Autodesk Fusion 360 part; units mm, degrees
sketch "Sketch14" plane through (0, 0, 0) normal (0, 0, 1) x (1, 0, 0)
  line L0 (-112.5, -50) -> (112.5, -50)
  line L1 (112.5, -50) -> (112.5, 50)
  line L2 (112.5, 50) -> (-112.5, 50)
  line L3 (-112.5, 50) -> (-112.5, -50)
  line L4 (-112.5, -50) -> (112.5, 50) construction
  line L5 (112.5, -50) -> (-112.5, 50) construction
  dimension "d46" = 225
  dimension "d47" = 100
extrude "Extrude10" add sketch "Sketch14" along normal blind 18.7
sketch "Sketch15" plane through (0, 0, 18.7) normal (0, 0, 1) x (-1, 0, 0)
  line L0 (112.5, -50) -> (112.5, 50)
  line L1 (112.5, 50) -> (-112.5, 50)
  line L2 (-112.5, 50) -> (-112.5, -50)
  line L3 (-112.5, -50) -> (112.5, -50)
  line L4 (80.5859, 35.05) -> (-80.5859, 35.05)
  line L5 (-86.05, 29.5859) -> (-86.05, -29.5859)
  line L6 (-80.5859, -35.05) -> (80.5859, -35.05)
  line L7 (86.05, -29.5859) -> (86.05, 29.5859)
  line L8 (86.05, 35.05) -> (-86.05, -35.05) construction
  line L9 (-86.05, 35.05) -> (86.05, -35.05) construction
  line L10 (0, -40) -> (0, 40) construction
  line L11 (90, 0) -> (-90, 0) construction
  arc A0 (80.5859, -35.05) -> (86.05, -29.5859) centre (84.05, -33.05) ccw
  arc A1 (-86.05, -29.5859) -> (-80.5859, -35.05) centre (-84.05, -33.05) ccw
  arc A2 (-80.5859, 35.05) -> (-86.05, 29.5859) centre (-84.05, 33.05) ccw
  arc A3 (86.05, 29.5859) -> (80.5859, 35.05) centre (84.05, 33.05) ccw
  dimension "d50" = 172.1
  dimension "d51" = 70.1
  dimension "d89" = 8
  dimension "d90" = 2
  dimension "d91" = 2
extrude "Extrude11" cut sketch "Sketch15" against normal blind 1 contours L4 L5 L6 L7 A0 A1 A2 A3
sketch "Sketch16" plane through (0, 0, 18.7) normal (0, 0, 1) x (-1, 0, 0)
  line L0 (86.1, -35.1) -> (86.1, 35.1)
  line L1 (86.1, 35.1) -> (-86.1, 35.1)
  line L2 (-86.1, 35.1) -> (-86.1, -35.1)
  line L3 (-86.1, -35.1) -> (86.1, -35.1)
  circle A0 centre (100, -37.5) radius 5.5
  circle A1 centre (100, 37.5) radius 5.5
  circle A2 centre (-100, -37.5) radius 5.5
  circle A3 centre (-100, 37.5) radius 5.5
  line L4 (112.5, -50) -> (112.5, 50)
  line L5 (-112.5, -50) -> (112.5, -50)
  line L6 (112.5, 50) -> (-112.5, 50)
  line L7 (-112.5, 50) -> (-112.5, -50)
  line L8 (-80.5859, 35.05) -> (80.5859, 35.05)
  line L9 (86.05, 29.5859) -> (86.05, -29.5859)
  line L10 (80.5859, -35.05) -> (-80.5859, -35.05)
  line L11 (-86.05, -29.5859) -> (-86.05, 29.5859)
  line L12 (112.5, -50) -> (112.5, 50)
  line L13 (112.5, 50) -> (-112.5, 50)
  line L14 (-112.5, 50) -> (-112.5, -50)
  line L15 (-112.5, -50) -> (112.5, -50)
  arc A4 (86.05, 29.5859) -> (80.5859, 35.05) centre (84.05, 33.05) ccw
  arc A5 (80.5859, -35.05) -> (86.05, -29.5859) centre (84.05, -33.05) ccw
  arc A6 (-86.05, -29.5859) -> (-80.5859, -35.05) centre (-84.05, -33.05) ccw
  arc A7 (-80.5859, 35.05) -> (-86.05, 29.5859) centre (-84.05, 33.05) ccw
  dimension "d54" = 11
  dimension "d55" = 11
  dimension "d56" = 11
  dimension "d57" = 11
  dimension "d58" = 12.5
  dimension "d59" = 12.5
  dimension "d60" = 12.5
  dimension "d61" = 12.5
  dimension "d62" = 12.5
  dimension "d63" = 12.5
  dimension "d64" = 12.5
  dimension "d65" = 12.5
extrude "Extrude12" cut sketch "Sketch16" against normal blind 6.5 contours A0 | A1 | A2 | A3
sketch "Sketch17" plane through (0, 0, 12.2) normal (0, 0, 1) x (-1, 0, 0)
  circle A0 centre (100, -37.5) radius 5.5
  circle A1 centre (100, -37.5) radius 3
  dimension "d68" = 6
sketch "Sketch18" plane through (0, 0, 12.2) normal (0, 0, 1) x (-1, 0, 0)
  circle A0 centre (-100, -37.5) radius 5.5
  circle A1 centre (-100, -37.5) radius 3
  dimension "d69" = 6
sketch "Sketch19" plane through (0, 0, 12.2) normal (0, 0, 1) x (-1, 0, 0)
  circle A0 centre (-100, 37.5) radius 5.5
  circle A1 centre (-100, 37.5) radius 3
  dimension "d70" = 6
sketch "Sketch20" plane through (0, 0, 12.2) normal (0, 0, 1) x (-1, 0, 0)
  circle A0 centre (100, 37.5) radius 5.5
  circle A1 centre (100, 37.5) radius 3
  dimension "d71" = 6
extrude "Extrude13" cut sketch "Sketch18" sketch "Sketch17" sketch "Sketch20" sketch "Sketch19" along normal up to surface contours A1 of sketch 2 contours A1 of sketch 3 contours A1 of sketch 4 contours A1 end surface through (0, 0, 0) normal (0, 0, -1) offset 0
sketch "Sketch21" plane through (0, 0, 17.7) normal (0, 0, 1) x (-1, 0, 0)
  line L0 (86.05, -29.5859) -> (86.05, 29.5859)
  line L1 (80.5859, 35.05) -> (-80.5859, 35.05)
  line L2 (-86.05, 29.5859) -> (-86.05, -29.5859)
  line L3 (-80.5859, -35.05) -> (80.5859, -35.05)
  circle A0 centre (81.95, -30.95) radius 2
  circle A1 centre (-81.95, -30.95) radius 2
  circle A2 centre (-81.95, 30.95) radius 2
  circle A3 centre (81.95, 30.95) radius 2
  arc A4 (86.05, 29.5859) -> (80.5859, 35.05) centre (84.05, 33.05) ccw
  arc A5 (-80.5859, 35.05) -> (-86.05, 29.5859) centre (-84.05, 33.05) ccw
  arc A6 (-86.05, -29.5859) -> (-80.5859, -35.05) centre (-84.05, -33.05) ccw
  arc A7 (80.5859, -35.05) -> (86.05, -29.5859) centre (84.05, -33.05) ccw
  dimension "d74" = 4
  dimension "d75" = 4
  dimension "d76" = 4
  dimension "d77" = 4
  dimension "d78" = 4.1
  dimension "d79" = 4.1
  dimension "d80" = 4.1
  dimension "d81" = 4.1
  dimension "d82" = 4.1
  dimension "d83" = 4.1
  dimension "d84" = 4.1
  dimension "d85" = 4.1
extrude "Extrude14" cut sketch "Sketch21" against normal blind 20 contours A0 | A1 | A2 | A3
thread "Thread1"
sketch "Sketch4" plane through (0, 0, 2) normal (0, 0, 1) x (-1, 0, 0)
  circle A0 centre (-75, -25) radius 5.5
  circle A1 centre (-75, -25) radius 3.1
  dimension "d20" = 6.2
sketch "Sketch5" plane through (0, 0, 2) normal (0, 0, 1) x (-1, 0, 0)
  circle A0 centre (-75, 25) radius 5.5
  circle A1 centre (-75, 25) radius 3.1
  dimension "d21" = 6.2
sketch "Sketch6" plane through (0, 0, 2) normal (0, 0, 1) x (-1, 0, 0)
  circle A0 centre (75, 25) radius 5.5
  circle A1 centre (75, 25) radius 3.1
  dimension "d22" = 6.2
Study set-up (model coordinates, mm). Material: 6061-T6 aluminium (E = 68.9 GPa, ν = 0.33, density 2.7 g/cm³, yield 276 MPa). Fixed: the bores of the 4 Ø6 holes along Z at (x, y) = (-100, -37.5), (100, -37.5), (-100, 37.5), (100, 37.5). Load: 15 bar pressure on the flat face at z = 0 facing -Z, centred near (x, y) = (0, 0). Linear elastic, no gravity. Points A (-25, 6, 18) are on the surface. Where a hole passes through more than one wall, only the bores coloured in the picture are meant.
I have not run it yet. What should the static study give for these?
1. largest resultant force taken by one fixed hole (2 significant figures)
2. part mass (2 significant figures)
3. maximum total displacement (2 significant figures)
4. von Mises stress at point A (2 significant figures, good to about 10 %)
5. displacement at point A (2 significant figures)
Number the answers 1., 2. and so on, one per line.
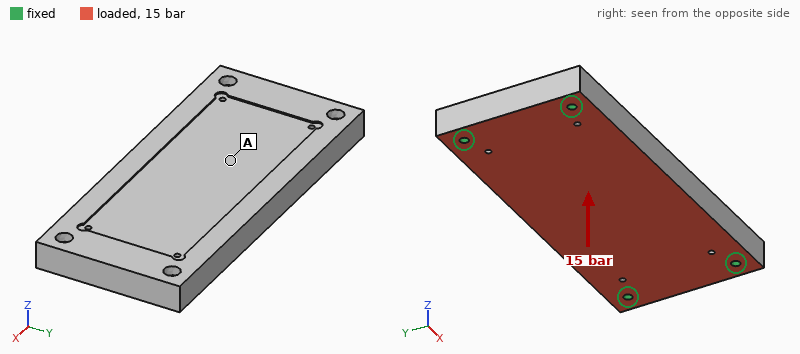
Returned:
1. 9.5 kN
2. 1.1 kg
3. 0.37 mm
4. 54 MPa
5. 0.32 mm
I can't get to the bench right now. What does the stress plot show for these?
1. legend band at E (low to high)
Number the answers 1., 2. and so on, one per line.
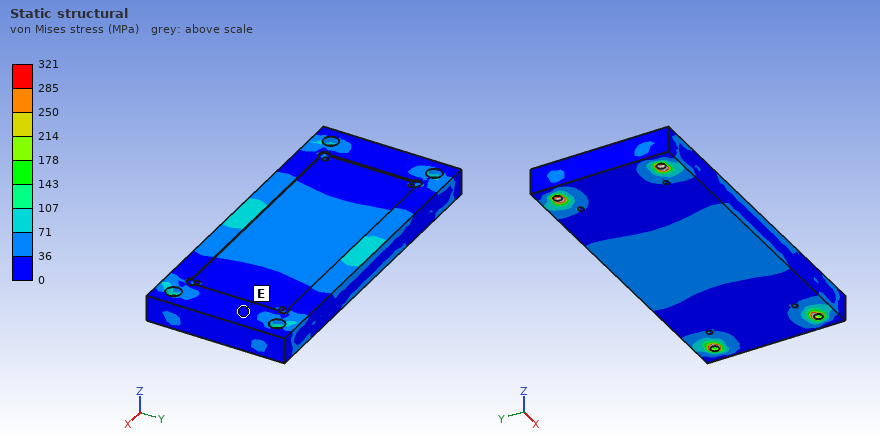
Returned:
1. 0 to 36 MPa
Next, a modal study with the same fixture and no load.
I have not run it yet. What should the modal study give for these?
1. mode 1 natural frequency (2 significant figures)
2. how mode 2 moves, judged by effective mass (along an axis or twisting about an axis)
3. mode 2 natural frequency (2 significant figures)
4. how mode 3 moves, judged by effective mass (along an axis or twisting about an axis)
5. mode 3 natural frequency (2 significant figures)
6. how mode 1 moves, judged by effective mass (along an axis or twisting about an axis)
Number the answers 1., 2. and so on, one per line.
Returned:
1. 1700 Hz
2. twisting about X
3. 3100 Hz
4. twisting about Y
5. 4600 Hz
6. along Z
